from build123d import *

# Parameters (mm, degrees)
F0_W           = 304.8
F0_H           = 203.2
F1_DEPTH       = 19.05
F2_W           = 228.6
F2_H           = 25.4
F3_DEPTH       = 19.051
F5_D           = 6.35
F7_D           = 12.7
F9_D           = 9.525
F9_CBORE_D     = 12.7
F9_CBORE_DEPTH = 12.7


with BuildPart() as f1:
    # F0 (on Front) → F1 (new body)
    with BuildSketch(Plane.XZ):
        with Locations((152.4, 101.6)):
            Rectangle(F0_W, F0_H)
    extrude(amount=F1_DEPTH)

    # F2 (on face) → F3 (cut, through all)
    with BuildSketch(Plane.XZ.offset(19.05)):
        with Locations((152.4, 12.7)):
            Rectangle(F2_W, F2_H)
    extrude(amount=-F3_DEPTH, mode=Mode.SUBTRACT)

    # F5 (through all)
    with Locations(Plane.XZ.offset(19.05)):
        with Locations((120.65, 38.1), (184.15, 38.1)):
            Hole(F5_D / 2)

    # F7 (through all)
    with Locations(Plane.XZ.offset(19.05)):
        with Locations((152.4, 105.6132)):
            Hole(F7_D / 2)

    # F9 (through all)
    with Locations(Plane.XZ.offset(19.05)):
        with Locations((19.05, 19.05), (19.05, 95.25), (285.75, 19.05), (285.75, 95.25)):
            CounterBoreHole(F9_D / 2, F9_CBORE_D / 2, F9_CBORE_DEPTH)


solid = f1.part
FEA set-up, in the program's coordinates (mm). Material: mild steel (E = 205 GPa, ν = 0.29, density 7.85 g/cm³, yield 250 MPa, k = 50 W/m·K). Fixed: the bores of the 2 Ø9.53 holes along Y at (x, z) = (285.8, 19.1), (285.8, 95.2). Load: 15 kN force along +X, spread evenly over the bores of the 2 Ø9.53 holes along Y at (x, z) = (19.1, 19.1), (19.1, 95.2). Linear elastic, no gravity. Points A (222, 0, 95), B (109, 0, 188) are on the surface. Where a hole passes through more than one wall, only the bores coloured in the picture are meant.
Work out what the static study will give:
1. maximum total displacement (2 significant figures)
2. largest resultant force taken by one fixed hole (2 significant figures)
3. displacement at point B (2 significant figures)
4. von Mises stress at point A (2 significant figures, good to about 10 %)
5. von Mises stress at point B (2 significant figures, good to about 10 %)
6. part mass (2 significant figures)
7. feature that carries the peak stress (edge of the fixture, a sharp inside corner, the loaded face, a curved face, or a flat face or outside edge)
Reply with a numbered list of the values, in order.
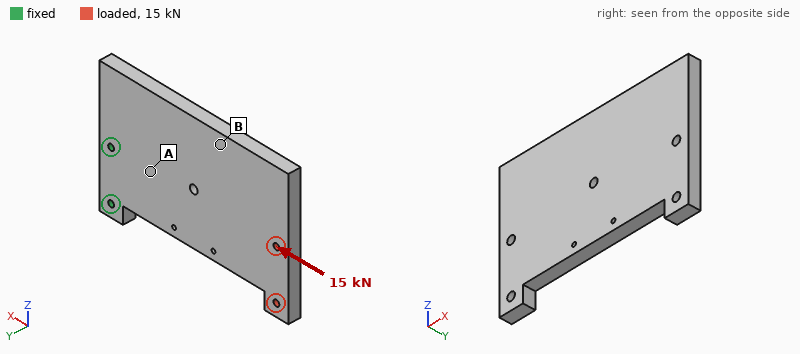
1. 0.23 mm
2. 7.7 kN
3. 0.092 mm
4. 15 MPa
5. 5.2 MPa
6. 8.3 kg
7. edge of the fixture
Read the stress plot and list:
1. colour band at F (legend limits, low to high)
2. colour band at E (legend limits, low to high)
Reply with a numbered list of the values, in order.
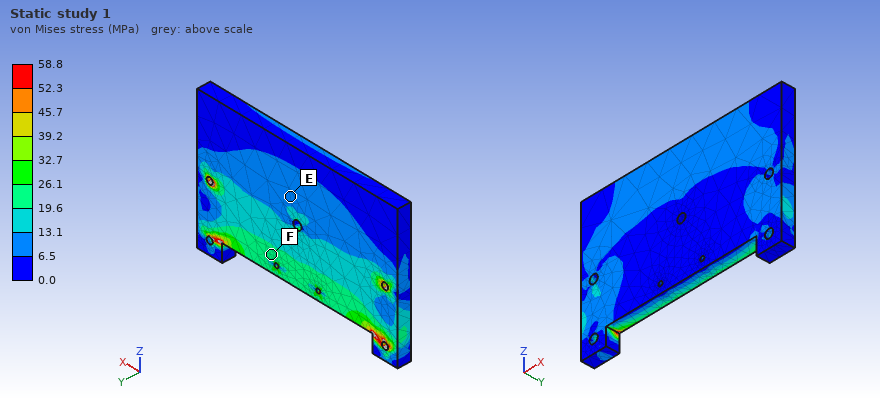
1. 19.6 to 26.1 MPa
2. 6.5 to 13.1 MPa
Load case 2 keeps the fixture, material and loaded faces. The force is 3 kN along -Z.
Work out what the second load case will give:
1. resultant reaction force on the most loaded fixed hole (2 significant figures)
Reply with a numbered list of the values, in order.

1. 10 kN
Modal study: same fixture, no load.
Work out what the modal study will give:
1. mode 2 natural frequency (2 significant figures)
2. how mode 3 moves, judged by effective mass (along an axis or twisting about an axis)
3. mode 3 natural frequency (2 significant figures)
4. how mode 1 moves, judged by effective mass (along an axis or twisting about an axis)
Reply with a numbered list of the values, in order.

1. 450 Hz
2. along Z
3. 580 Hz
4. along Y
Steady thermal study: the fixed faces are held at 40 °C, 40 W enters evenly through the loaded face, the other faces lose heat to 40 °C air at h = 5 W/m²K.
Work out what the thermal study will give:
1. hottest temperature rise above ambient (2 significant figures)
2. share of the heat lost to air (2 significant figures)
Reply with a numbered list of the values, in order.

1. 80 K
2. 48 %
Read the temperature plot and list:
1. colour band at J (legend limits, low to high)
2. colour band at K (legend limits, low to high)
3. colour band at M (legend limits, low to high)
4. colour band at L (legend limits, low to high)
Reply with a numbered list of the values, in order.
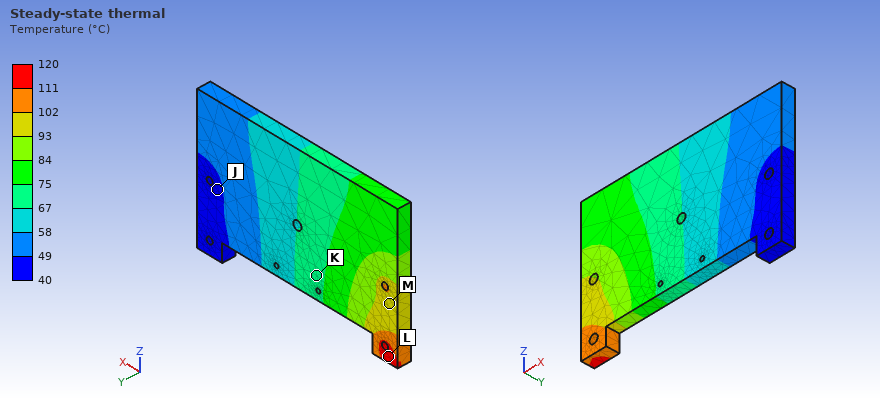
1. 40 to 49 °C
2. 67 to 75 °C
3. 93 to 102 °C
4. 111 to 120 °C
